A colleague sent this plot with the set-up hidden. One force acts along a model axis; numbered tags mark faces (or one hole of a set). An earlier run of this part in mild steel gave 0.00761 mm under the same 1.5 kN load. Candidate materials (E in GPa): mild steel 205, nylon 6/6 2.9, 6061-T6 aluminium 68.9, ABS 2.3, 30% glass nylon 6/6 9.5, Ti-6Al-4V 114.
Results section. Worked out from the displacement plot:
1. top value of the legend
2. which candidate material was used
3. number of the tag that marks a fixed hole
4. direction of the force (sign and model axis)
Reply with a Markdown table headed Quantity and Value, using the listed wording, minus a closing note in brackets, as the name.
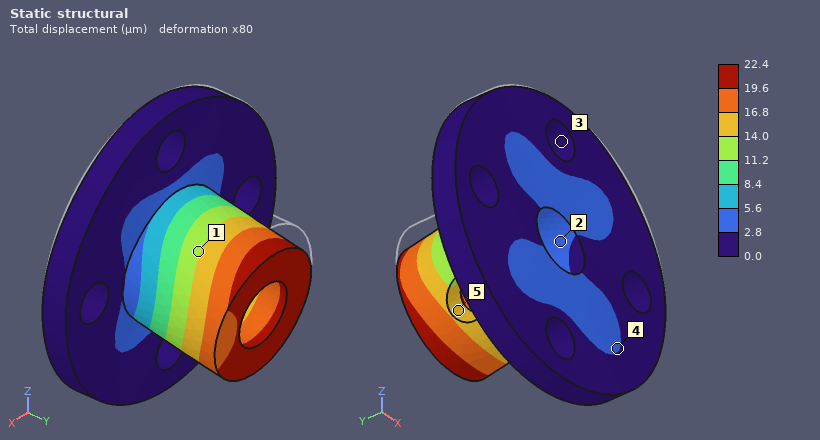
| Quantity | Value |
|---|---|
| top value of the legend | 22.4 µm |
| which candidate material was used | 6061-T6 aluminium |
| number of the tag that marks a fixed hole | 3 |
| direction of the force | -Z |
